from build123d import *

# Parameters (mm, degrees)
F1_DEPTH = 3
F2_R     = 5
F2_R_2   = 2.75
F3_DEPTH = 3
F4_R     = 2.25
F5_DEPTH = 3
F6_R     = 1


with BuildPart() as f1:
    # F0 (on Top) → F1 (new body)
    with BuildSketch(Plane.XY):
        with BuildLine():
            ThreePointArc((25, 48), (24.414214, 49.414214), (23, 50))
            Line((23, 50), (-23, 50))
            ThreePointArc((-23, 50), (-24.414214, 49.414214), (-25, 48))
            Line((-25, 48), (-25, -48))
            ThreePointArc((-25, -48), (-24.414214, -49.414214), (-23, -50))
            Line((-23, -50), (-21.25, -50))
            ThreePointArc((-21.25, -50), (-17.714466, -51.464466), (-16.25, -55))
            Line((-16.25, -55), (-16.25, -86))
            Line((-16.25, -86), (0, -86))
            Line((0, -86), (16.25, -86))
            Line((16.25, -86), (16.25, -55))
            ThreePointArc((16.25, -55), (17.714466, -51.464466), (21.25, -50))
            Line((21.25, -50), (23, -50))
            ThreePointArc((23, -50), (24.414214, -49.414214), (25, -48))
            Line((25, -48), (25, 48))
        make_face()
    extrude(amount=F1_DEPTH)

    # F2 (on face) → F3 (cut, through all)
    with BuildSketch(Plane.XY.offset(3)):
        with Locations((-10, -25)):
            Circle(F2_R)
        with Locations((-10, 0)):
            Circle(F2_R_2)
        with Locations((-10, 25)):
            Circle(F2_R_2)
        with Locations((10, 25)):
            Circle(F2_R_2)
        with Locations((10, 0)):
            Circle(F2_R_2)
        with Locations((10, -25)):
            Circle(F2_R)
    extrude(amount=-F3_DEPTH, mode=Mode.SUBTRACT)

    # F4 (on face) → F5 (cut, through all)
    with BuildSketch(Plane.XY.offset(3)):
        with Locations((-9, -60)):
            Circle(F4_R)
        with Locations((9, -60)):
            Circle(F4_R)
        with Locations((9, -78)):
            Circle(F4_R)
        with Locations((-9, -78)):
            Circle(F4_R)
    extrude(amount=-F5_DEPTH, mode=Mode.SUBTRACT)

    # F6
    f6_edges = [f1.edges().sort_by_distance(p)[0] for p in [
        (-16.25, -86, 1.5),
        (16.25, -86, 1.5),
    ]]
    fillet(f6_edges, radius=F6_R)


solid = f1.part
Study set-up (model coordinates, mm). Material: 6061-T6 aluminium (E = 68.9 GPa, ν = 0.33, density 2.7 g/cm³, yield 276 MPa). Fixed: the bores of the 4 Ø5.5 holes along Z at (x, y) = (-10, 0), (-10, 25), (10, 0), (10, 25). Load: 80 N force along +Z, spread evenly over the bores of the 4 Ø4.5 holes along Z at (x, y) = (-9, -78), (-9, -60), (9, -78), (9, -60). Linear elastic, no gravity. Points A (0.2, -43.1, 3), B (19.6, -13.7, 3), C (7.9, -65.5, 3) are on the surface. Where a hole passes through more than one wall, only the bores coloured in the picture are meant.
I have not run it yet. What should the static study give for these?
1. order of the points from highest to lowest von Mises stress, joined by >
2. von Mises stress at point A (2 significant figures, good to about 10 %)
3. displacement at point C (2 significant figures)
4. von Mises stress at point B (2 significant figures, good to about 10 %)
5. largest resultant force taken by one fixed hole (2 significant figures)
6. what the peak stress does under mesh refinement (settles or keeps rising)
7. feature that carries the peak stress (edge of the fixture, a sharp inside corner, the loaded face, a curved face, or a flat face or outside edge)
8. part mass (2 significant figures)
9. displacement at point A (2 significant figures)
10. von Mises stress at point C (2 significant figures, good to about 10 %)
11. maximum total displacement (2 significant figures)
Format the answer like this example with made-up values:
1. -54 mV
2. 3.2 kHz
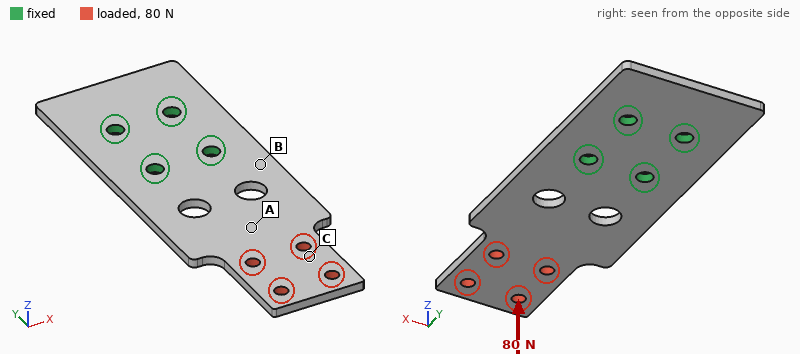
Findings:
1. B > A > C
2. 29 MPa
3. 1.1 mm
4. 60 MPa
5. 56 N
6. keeps rising
7. edge of the fixture
8. 47 g
9. 0.55 mm
10. 13 MPa
11. 1.7 mm
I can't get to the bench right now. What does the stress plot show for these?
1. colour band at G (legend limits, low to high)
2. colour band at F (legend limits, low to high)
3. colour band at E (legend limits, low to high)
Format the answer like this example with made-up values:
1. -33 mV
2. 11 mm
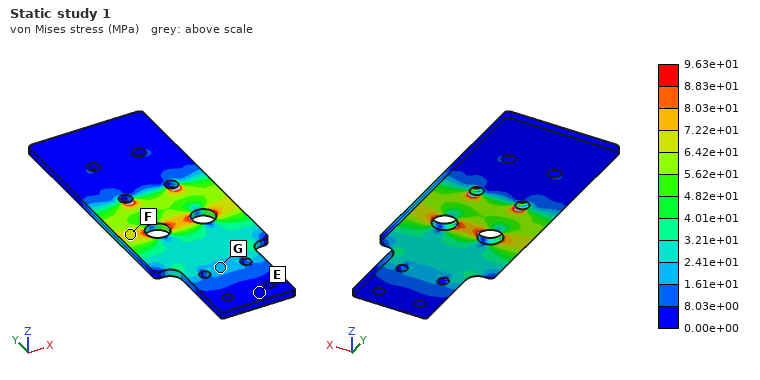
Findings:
1. 1.61e+01 to 2.41e+01 MPa
2. 6.42e+01 to 7.22e+01 MPa
3. 0.00e+00 to 8.03e+00 MPa
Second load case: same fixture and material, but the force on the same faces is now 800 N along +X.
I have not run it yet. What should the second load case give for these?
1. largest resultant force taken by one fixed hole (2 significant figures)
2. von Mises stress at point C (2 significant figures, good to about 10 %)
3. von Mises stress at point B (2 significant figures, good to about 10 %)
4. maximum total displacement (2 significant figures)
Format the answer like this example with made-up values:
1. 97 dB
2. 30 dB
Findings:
1. 1.5 kN
2. 10 MPa
3. 29 MPa
4. 0.12 mm
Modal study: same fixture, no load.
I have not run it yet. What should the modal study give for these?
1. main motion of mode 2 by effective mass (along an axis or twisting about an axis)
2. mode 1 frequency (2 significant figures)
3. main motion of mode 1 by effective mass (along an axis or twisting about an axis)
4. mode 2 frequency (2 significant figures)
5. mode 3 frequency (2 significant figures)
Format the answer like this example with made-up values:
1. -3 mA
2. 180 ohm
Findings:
1. twisting about Y
2. 400 Hz
3. along Z
4. 1700 Hz
5. 2100 Hz
